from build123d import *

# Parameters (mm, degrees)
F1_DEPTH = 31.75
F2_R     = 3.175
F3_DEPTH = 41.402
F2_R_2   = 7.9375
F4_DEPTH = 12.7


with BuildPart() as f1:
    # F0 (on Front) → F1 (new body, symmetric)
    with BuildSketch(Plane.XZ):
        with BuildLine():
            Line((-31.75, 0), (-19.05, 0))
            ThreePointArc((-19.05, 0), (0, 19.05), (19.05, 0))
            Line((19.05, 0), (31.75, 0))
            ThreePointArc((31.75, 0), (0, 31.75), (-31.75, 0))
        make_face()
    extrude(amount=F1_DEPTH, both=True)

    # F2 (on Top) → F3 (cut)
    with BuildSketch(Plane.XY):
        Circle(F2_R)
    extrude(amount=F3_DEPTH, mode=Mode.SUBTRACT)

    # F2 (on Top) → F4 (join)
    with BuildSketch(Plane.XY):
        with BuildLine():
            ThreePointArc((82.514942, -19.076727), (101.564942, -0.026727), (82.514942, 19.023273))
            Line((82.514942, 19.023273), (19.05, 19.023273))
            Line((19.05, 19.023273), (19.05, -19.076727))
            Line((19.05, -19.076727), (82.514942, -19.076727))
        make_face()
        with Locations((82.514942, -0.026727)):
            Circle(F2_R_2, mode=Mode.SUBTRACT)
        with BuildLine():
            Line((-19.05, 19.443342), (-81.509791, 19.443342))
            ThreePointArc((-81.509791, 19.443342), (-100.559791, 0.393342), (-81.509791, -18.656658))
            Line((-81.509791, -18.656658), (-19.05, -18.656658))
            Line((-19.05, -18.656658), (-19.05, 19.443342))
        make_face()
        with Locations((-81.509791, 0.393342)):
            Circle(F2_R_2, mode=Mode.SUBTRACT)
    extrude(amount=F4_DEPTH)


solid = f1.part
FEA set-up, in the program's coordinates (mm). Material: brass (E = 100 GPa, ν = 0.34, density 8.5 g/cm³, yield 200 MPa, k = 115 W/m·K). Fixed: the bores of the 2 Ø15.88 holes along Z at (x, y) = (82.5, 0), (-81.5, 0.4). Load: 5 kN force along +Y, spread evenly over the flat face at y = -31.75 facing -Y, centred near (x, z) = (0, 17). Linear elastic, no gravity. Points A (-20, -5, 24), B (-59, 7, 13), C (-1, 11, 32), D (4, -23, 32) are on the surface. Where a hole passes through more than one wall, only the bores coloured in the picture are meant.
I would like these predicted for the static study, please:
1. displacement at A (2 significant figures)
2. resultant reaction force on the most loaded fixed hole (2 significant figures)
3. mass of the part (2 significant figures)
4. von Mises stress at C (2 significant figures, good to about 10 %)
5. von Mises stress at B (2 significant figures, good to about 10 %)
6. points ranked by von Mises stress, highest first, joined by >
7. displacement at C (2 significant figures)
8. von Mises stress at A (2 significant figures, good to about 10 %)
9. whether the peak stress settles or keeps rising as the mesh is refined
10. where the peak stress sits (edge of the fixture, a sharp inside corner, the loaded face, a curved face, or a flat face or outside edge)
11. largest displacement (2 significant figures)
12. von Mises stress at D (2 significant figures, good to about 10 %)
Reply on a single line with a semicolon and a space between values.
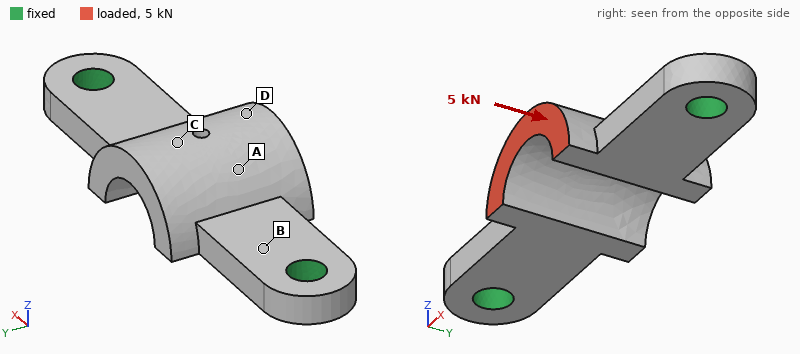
0.063 mm; 2.5 kN; 1.0 kg; 4.9 MPa; 35 MPa; B > A > D > C; 0.081 mm; 17 MPa; keeps rising; edge of the fixture; 0.10 mm; 12 MPa
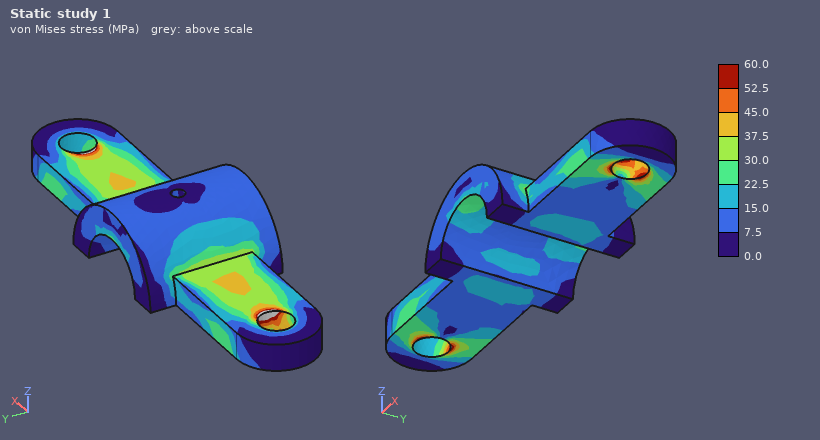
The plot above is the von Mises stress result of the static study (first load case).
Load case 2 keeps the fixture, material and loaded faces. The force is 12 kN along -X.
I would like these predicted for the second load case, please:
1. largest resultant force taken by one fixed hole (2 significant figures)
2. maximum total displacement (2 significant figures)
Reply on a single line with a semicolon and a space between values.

6.8 kN; 44 µm
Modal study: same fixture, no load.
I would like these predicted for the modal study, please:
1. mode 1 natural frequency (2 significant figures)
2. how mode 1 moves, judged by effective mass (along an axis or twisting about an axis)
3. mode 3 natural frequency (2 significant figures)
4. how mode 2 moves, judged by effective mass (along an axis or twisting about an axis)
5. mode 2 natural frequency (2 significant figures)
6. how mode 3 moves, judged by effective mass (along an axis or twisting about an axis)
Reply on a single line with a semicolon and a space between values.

1600 Hz; along Y; 3200 Hz; along Z; 1700 Hz; along Y
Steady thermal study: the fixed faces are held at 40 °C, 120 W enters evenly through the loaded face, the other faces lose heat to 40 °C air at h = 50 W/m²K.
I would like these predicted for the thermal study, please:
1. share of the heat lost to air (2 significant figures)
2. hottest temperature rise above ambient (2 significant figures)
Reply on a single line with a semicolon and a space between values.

30 %; 70 K
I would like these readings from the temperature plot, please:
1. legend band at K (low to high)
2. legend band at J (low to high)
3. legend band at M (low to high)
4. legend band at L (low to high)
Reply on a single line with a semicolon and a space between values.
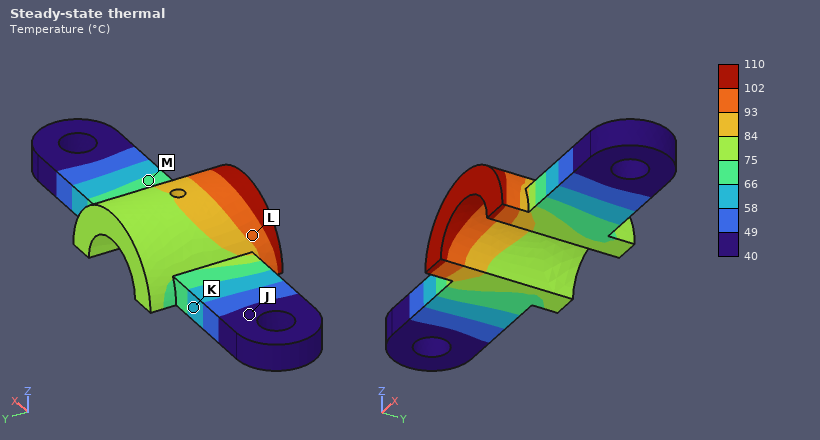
58 to 66 °C; 40 to 49 °C; 66 to 75 °C; 93 to 102 °C
